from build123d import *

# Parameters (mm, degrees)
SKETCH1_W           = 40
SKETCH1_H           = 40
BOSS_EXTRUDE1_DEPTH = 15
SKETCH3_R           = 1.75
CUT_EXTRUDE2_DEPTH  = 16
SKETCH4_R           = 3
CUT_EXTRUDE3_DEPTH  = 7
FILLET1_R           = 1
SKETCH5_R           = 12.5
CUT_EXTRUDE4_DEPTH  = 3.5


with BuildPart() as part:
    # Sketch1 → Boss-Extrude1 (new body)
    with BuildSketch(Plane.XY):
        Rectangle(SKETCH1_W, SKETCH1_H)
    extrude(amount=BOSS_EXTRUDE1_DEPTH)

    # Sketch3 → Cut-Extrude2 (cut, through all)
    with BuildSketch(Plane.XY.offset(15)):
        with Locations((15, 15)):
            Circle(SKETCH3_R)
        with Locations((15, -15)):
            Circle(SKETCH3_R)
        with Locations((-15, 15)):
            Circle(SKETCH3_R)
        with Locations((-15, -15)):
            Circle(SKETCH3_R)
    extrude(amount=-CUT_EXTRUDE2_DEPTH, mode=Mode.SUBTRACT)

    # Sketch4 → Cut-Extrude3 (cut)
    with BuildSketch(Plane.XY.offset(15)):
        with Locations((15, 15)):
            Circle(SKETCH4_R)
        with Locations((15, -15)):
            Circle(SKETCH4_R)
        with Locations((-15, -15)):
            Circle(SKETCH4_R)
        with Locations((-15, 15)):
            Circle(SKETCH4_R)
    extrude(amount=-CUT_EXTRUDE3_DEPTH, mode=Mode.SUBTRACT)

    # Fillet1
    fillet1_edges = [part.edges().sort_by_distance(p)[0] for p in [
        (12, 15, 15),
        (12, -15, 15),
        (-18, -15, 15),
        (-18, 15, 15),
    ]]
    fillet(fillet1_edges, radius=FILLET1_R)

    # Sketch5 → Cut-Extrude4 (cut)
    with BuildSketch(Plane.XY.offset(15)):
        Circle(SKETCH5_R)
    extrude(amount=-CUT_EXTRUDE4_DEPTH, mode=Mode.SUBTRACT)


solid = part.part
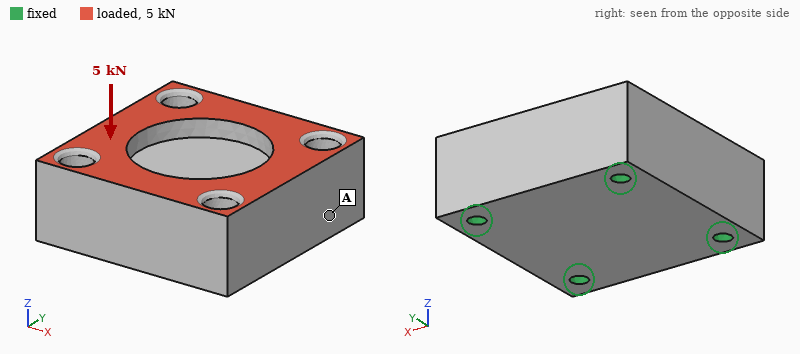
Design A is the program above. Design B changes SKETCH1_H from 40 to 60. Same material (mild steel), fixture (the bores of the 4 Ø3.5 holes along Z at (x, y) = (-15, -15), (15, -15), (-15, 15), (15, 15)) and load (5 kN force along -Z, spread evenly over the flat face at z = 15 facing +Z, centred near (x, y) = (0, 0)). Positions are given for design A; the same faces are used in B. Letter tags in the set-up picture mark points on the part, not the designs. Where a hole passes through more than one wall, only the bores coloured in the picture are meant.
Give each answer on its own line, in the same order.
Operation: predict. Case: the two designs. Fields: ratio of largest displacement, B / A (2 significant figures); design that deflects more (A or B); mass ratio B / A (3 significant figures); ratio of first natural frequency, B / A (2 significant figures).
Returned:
2.1
B
1.57
0.71
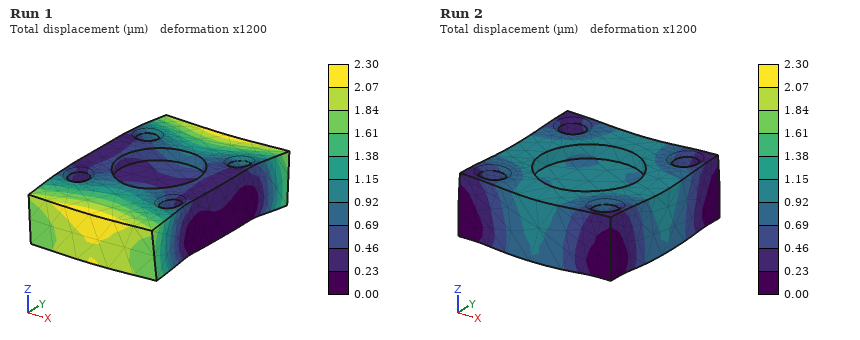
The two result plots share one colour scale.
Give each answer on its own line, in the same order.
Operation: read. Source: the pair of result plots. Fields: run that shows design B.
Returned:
Run 1
